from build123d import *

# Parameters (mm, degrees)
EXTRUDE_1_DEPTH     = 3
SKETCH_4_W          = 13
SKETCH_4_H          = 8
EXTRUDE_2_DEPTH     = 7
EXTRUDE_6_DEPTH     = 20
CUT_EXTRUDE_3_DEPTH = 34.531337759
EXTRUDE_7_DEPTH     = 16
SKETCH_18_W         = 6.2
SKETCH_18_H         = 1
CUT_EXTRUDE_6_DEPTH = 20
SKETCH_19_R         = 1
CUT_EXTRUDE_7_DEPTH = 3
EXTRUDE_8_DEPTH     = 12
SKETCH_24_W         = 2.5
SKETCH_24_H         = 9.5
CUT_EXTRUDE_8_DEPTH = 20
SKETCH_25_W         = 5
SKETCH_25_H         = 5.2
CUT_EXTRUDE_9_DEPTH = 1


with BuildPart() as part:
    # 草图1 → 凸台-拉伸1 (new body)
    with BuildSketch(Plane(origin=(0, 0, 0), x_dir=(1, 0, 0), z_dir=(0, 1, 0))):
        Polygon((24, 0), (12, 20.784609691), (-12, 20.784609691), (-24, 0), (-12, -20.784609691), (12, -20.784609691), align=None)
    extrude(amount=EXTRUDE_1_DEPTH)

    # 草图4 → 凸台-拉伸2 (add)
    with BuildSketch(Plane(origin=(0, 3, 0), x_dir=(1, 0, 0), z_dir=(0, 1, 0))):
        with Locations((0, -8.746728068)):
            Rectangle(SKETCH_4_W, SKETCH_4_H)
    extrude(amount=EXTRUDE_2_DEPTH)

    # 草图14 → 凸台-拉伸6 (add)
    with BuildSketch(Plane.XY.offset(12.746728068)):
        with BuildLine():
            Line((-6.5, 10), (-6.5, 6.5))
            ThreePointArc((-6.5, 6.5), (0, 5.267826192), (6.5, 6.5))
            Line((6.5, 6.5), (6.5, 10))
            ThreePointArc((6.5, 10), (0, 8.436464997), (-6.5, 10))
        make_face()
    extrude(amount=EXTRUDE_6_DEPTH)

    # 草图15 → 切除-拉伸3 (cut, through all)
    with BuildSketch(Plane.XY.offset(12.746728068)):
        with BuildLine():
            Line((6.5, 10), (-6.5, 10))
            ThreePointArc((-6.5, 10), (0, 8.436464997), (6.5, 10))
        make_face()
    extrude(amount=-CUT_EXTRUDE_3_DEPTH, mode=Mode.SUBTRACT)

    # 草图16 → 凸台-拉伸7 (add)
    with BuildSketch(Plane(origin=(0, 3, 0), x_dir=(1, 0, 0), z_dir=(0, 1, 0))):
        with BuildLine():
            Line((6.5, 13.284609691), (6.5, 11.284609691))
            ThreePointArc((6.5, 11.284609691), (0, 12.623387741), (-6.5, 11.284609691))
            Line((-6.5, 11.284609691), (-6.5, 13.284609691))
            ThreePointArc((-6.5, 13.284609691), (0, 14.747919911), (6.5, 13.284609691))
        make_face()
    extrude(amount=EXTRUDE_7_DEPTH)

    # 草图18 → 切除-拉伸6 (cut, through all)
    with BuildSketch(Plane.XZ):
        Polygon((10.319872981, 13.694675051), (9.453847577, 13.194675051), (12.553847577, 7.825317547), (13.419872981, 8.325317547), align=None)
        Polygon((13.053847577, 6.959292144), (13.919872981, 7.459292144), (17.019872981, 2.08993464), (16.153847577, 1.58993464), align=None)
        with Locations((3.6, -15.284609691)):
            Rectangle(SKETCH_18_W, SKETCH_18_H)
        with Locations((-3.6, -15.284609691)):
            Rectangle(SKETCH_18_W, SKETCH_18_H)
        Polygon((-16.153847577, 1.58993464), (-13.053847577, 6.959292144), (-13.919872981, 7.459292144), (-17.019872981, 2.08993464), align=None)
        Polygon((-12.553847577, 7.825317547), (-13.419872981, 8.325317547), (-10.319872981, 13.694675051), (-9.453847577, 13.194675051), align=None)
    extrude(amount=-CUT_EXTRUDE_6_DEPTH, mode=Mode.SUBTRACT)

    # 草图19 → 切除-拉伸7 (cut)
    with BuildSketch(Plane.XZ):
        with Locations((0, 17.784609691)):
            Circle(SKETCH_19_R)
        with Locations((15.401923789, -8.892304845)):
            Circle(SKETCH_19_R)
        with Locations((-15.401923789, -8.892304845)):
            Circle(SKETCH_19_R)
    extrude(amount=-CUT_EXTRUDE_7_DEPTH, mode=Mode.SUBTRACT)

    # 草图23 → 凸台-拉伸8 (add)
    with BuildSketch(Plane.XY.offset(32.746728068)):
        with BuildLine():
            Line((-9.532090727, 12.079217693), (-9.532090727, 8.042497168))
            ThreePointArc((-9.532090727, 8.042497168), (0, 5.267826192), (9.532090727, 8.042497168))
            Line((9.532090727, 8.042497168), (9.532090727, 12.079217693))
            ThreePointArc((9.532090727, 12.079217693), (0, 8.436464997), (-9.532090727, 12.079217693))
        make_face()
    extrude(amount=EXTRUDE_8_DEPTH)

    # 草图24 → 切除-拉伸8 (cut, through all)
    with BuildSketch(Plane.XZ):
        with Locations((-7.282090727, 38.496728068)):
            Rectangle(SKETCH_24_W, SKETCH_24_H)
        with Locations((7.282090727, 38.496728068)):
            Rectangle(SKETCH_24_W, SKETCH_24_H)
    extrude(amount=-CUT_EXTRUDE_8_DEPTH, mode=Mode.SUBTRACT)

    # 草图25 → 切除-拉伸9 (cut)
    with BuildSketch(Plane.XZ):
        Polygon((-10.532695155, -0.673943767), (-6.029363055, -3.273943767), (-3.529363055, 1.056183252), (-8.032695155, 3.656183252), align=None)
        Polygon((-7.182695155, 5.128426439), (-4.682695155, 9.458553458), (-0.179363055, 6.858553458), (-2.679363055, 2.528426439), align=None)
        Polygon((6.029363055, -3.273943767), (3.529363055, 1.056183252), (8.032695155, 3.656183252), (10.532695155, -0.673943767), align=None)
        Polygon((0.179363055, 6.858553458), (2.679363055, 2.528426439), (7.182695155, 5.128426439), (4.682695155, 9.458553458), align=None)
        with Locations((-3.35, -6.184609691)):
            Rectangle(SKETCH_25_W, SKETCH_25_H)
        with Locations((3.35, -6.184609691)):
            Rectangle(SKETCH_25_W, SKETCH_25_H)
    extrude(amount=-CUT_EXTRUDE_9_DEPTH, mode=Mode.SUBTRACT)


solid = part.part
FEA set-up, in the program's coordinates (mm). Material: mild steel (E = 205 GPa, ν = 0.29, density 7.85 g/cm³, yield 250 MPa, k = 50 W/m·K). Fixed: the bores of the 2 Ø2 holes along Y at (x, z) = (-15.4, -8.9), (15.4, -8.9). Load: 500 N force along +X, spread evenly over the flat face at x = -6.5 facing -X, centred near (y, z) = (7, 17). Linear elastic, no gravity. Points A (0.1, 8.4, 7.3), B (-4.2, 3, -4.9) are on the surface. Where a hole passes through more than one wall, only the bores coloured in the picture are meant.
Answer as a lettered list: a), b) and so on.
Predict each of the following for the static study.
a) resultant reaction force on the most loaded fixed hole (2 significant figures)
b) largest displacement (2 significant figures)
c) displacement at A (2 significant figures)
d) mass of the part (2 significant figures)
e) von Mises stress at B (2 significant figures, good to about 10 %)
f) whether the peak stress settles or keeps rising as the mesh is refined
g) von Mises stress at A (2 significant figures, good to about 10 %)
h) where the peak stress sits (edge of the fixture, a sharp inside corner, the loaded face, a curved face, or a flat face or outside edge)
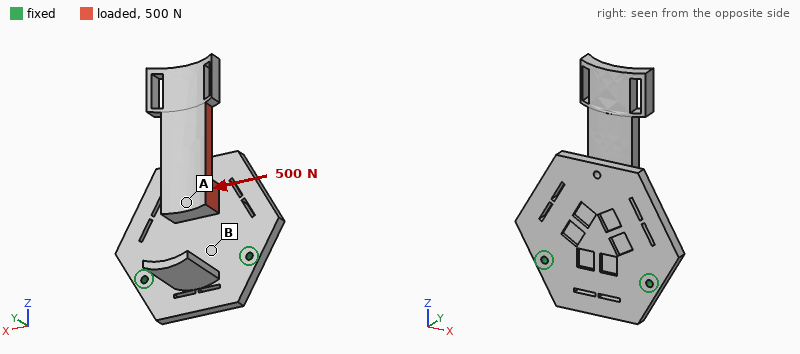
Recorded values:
a) 490 N
b) 32 µm
c) 8.3 µm
d) 53 g
e) 24 MPa
f) keeps rising
g) 8.3 MPa
h) edge of the fixture
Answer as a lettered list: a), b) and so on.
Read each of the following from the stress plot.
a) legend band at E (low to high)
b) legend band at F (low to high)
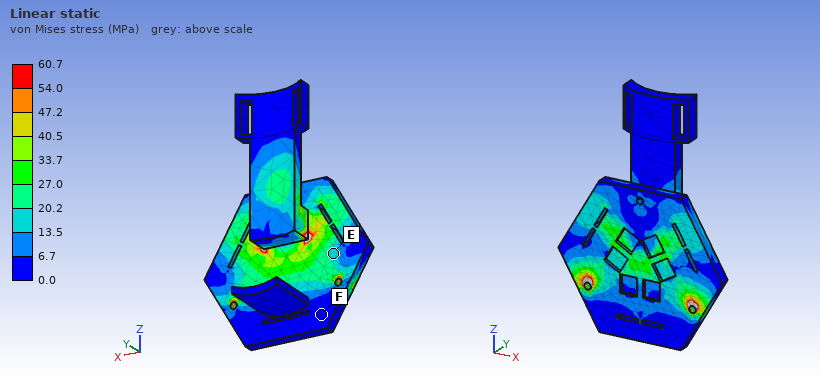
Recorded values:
a) 13.5 to 20.2 MPa
b) 0.0 to 6.7 MPa
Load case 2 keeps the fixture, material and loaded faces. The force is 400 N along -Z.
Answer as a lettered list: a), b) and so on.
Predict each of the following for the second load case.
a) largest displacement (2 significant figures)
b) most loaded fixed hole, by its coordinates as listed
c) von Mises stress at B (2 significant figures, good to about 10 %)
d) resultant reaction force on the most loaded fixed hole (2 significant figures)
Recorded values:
a) 0.15 mm
b) (-15.4, -8.9)
c) 34 MPa
d) 290 N
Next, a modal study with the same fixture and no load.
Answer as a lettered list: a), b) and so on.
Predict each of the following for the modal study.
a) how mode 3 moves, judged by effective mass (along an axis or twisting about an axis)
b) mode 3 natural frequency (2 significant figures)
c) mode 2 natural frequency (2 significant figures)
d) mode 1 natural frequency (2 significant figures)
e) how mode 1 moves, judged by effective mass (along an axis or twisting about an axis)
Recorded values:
a) along X
b) 4900 Hz
c) 3900 Hz
d) 1000 Hz
e) along Y
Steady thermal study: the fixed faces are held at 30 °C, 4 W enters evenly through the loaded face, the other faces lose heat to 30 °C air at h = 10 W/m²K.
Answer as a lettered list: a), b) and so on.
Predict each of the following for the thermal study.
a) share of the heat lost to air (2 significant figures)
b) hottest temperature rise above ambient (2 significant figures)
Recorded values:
a) 18 %
b) 31 K
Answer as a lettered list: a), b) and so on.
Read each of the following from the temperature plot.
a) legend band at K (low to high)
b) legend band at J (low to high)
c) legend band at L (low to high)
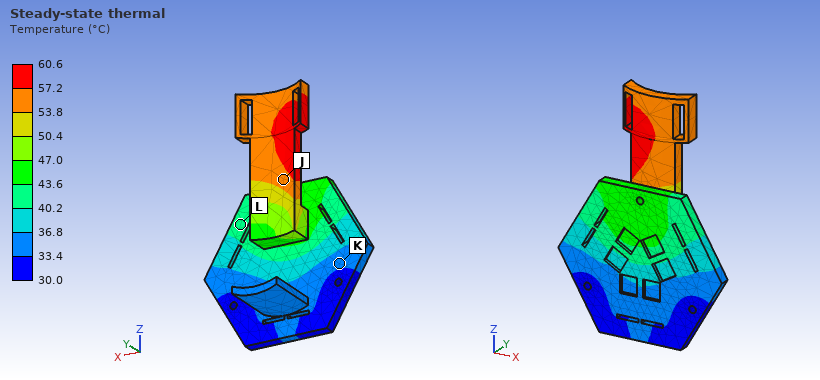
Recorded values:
a) 33.4 to 36.8 °C
b) 53.8 to 57.2 °C
c) 40.2 to 43.6 °C
